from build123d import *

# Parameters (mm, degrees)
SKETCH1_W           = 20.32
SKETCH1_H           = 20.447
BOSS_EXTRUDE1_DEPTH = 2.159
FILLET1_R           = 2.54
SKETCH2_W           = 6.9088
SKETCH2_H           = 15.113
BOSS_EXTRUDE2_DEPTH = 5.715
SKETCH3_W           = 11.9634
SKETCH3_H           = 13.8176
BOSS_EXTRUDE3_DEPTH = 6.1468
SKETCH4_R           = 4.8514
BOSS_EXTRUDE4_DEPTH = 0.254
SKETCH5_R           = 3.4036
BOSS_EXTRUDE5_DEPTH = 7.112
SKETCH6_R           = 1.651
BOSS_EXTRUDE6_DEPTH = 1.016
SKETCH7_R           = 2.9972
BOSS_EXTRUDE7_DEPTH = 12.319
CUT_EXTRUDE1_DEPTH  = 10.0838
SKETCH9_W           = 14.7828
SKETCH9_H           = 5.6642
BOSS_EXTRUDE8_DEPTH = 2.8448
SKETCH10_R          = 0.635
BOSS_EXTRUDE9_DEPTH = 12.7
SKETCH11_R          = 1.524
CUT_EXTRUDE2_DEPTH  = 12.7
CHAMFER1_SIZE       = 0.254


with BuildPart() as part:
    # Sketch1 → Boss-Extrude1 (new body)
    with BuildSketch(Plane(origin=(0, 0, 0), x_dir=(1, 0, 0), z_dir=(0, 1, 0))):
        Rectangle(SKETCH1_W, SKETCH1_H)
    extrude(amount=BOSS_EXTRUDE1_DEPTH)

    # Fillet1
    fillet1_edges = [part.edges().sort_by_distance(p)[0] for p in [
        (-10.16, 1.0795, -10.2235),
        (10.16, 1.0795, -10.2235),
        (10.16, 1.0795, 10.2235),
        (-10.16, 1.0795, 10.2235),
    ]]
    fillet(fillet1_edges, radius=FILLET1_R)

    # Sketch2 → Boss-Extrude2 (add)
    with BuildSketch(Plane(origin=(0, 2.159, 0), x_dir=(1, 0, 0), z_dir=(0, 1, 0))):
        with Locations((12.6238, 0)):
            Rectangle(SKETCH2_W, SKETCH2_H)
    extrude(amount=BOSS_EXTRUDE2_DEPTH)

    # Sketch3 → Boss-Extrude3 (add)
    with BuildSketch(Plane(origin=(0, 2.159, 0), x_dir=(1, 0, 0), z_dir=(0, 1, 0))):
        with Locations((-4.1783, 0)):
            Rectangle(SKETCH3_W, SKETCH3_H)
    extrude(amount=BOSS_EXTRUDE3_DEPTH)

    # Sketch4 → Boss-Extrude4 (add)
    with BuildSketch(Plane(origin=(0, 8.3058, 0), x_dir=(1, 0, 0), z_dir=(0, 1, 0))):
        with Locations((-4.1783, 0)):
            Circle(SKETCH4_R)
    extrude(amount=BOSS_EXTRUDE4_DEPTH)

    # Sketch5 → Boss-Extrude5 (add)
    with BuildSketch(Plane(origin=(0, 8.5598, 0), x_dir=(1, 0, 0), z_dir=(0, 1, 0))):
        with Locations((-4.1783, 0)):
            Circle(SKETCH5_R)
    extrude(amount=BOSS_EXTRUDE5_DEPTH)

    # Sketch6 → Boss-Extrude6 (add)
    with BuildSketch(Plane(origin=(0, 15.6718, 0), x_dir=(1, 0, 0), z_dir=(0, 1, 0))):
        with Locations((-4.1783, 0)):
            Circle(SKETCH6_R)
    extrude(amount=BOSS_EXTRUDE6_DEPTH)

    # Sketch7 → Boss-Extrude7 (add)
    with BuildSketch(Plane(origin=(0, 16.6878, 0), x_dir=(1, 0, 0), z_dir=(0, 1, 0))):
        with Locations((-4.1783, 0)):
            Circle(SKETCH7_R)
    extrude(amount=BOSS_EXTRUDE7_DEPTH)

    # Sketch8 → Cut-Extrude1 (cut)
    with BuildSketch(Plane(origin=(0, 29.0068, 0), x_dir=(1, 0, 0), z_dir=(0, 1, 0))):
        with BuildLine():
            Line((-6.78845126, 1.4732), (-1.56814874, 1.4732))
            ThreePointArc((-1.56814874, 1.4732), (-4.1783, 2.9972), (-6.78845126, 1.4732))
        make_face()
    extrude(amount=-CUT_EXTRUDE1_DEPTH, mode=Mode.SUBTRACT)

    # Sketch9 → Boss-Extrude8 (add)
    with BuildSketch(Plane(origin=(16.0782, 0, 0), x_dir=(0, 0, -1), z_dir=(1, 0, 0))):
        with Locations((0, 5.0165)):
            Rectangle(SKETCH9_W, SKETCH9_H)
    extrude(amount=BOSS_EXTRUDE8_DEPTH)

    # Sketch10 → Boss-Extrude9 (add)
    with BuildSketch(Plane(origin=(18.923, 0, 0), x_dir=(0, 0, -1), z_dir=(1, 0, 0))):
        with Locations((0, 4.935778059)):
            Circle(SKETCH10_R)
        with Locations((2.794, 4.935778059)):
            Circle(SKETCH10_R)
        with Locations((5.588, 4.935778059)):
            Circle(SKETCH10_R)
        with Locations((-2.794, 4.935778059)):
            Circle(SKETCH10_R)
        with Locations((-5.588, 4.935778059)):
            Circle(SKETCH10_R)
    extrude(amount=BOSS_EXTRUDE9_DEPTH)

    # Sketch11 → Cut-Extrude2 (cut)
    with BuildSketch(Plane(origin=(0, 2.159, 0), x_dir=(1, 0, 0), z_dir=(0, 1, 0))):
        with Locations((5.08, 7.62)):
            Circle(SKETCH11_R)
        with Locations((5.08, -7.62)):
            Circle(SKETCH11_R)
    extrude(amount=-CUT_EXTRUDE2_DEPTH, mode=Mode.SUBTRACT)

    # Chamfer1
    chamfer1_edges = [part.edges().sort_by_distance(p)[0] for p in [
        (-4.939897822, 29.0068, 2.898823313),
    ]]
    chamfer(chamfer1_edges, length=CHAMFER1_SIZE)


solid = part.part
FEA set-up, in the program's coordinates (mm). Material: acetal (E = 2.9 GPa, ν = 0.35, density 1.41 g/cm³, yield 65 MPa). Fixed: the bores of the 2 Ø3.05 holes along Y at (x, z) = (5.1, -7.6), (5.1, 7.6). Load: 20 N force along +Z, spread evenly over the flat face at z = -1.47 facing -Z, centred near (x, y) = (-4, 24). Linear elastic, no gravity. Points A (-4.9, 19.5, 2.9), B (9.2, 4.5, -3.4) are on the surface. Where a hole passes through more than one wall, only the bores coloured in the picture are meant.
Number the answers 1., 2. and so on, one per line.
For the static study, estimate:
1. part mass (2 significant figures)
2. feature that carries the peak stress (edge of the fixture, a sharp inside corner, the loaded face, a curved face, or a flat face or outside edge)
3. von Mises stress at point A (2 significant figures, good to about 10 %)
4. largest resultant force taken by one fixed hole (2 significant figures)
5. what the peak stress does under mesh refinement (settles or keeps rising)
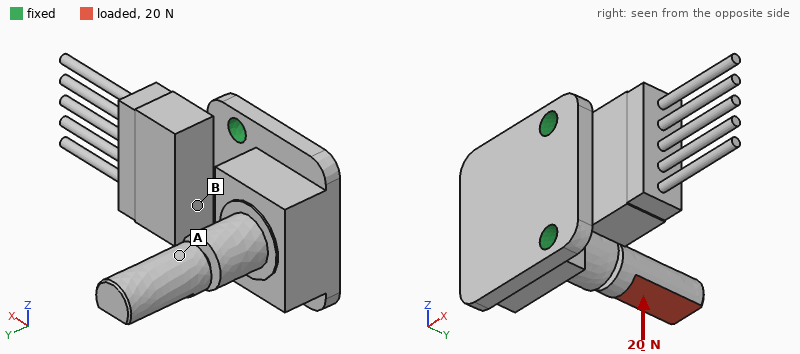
1. 4.7 g
2. a sharp inside corner
3. 5.3 MPa
4. 36 N
5. keeps rising
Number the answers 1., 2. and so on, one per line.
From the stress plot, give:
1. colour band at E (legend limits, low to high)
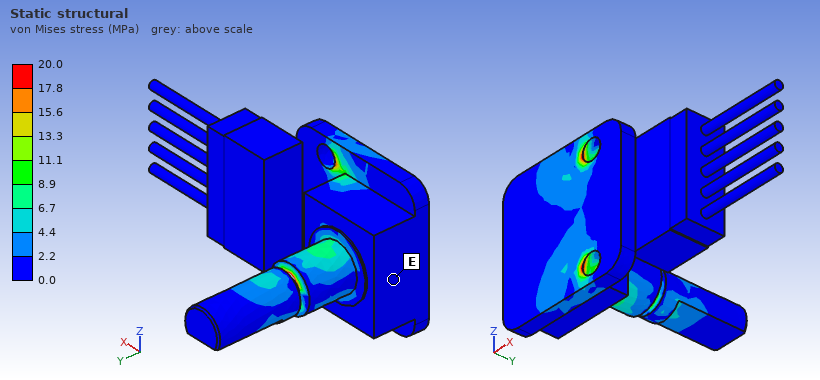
1. 0.0 to 2.2 MPa
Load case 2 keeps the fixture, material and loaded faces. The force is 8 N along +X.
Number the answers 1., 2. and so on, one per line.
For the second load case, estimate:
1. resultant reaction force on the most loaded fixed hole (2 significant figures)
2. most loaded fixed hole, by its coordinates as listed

1. 5.1 N
2. (5.1, -7.6)
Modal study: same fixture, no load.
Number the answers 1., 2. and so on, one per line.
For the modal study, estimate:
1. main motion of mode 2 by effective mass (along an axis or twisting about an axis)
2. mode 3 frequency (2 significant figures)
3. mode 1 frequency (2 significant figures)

1. along Y
2. 1500 Hz
3. 820 Hz
